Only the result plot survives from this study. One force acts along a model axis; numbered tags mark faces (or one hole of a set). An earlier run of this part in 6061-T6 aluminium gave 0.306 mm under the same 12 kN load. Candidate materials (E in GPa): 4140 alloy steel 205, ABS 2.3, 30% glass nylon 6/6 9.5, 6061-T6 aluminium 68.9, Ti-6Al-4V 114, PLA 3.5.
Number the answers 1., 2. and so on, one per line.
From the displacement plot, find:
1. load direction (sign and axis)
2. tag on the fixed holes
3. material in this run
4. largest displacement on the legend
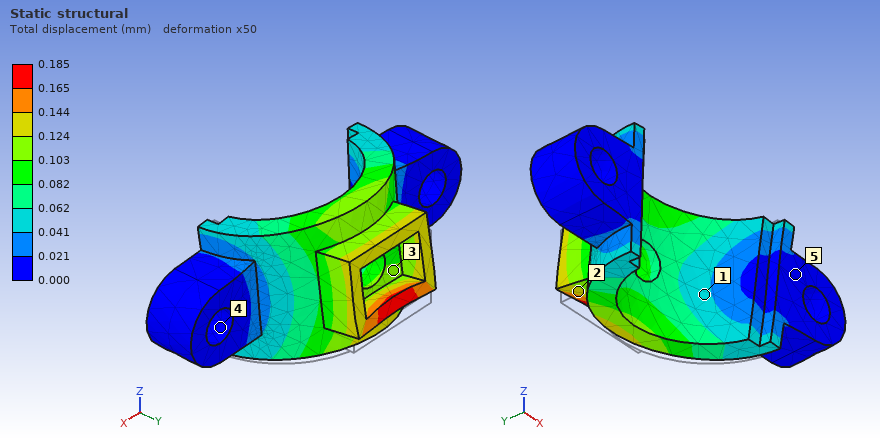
1. +Z
2. 4
3. Ti-6Al-4V
4. 0.185 mm
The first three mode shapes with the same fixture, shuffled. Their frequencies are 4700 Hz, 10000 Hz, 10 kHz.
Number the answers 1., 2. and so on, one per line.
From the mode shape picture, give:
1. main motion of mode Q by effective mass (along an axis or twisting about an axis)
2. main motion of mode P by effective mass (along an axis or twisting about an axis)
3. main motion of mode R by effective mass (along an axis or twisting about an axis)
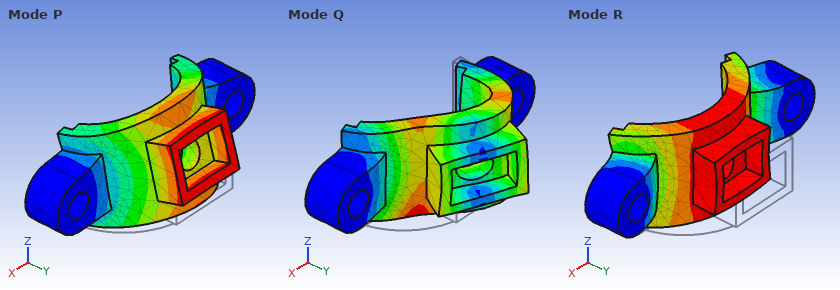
1. along X
2. along Z
3. along Y
